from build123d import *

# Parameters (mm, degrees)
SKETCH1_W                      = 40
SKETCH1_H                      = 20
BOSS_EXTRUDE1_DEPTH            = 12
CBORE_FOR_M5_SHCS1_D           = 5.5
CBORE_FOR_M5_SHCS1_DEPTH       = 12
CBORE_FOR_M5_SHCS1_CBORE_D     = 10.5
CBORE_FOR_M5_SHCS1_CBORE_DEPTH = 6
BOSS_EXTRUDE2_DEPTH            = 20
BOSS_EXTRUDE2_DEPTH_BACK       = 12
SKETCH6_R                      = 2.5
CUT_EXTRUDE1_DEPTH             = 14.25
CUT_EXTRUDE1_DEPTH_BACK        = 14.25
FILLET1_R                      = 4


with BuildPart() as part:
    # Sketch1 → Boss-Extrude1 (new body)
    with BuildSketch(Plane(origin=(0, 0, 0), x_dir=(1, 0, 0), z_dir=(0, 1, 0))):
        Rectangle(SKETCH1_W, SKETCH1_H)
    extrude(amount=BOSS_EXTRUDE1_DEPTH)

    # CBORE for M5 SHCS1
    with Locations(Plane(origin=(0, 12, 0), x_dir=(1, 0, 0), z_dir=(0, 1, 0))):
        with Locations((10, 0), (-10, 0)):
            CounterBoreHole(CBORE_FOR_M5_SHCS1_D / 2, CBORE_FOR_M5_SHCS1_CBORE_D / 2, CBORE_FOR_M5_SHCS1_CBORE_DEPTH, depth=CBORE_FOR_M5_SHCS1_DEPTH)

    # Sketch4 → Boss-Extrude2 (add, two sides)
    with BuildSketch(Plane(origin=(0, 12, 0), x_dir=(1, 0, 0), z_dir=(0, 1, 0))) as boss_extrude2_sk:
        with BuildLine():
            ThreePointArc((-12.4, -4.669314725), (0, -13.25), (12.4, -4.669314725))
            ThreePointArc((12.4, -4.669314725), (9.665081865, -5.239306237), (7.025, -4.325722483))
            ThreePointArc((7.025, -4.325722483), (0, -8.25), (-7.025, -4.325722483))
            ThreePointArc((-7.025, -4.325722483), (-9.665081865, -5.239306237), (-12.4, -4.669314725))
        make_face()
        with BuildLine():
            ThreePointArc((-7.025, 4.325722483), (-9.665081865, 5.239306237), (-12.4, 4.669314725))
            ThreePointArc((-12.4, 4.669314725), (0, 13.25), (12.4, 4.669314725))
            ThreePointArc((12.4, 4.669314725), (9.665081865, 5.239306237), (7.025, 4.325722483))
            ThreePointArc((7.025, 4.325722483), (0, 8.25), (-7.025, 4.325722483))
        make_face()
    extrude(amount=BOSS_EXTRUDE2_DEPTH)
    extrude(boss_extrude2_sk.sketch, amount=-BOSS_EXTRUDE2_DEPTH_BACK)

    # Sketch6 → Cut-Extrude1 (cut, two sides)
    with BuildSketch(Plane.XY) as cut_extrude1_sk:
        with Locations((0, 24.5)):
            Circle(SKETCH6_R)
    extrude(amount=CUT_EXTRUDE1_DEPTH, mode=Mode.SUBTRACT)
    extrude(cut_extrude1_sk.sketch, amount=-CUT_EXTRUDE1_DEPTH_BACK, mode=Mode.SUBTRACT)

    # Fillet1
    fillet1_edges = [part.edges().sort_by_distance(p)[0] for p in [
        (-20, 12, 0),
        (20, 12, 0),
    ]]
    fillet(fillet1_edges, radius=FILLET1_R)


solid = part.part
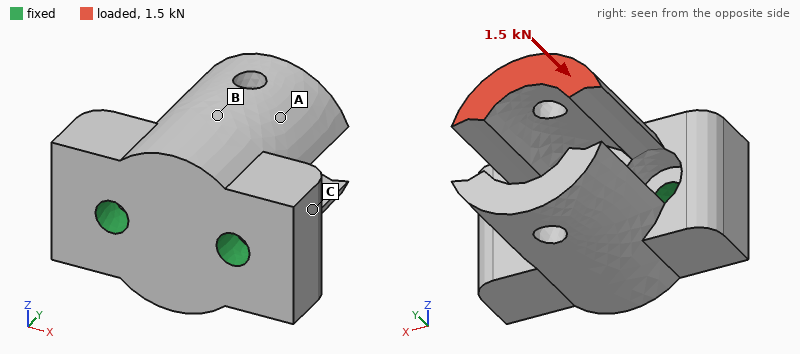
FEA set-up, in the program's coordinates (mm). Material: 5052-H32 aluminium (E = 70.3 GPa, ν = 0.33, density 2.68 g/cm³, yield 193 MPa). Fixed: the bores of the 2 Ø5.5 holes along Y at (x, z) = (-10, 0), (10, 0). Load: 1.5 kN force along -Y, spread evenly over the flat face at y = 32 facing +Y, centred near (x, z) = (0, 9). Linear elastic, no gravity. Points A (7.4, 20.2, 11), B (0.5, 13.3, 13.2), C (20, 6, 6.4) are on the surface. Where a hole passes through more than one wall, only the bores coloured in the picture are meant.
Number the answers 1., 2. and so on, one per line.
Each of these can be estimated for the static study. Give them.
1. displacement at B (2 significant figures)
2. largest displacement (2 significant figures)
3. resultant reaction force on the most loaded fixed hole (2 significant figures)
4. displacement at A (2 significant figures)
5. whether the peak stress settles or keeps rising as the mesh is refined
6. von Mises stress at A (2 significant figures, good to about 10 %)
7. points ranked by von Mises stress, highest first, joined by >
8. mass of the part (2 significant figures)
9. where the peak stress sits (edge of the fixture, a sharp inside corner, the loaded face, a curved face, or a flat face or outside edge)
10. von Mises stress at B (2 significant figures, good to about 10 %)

1. 14 µm
2. 32 µm
3. 780 N
4. 18 µm
5. keeps rising
6. 17 MPa
7. A > B > C
8. 36 g
9. edge of the fixture
10. 12 MPa
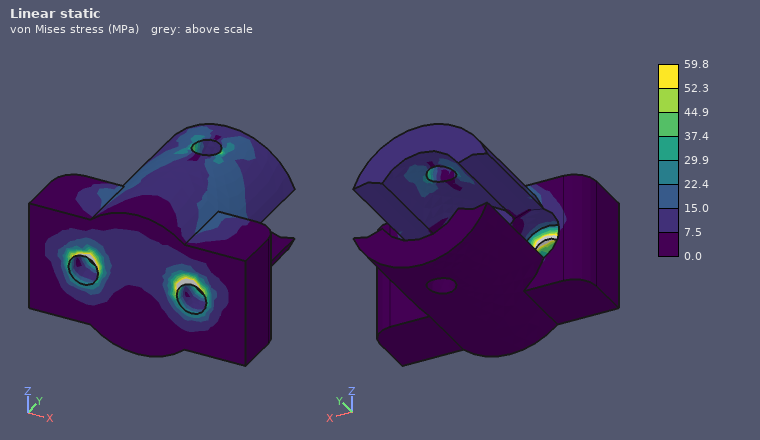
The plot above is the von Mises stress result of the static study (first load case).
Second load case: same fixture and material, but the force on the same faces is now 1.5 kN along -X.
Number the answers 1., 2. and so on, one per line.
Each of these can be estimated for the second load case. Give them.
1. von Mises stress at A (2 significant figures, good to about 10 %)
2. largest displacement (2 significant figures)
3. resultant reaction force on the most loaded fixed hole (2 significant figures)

1. 48 MPa
2. 93 µm
3. 2.1 kN
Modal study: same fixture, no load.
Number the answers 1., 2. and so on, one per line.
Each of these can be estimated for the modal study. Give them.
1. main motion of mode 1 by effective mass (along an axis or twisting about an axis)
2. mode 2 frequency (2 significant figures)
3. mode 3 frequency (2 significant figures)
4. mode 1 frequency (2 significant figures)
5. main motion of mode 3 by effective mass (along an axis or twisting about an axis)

1. along Z
2. 8700 Hz
3. 14 kHz
4. 6600 Hz
5. along X
